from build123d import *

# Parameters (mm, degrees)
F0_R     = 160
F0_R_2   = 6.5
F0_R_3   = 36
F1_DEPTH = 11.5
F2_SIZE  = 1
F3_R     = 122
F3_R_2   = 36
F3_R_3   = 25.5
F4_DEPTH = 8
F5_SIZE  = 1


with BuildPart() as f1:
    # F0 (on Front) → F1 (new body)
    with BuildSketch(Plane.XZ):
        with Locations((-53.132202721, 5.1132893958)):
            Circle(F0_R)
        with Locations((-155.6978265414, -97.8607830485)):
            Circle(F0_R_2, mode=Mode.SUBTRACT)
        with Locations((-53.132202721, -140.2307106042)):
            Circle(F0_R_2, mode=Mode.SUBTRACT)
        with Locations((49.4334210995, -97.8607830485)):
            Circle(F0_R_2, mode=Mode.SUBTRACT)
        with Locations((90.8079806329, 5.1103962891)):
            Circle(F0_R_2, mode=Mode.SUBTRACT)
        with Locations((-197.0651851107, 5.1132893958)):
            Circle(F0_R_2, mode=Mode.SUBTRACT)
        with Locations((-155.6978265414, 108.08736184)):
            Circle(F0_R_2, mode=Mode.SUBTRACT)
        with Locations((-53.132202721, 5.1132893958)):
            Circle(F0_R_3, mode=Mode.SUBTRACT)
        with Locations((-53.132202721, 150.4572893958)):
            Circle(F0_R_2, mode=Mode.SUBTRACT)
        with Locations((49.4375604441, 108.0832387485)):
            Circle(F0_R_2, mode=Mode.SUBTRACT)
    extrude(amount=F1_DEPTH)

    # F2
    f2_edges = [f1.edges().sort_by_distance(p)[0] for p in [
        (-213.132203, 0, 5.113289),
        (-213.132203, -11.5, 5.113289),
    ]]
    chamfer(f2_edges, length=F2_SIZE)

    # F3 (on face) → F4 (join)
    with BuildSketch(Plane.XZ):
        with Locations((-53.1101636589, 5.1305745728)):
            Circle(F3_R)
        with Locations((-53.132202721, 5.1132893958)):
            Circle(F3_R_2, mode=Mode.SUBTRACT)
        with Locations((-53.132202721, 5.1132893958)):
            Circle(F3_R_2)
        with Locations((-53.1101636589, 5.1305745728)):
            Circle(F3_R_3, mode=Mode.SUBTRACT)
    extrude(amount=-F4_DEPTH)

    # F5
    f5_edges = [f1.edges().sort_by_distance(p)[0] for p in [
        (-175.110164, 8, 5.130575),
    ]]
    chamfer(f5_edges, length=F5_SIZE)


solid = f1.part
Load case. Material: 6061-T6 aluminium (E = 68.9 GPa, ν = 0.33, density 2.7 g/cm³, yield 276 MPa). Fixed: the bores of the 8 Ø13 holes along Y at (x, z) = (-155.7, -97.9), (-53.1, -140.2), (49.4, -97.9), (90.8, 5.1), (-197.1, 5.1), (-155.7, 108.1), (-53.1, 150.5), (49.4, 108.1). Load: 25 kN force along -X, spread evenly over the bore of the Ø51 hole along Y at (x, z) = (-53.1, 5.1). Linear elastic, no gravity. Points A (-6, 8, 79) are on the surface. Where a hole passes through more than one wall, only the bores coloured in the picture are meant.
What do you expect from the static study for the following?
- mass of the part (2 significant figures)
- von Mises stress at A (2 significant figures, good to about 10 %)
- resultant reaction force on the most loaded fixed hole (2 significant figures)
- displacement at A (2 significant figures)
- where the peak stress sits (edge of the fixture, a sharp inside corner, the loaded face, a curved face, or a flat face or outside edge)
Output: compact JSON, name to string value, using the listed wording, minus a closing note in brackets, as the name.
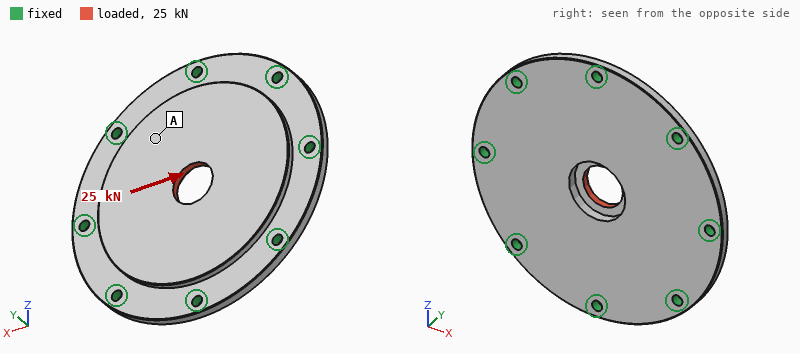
{"mass of the part": "3.3 kg", "von Mises stress at A": "3.1 MPa", "resultant reaction force on the most loaded fixed hole": "5.0 kN", "displacement at A": "4.8 µm", "where the peak stress sits": "a sharp inside corner"}
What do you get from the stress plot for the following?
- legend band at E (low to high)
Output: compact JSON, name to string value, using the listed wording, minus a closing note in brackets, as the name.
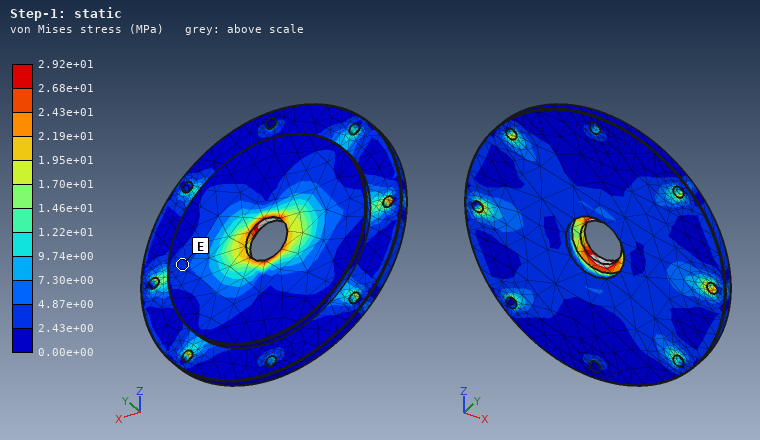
{"legend band at E": "2.43e+00 to 4.87e+00 MPa"}
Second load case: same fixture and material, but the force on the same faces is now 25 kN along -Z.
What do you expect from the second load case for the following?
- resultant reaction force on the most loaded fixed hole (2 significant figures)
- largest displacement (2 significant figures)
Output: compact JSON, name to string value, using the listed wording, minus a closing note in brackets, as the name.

{"resultant reaction force on the most loaded fixed hole": "4.9 kN", "largest displacement": "20 µm"}
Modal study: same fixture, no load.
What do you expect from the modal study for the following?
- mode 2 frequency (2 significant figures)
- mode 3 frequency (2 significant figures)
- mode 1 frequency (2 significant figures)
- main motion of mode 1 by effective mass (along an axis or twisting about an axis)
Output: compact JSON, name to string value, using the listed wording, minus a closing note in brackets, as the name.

{"mode 2 frequency": "3000 Hz", "mode 3 frequency": "3100 Hz", "mode 1 frequency": "1500 Hz", "main motion of mode 1 by effective mass": "along Y"}
